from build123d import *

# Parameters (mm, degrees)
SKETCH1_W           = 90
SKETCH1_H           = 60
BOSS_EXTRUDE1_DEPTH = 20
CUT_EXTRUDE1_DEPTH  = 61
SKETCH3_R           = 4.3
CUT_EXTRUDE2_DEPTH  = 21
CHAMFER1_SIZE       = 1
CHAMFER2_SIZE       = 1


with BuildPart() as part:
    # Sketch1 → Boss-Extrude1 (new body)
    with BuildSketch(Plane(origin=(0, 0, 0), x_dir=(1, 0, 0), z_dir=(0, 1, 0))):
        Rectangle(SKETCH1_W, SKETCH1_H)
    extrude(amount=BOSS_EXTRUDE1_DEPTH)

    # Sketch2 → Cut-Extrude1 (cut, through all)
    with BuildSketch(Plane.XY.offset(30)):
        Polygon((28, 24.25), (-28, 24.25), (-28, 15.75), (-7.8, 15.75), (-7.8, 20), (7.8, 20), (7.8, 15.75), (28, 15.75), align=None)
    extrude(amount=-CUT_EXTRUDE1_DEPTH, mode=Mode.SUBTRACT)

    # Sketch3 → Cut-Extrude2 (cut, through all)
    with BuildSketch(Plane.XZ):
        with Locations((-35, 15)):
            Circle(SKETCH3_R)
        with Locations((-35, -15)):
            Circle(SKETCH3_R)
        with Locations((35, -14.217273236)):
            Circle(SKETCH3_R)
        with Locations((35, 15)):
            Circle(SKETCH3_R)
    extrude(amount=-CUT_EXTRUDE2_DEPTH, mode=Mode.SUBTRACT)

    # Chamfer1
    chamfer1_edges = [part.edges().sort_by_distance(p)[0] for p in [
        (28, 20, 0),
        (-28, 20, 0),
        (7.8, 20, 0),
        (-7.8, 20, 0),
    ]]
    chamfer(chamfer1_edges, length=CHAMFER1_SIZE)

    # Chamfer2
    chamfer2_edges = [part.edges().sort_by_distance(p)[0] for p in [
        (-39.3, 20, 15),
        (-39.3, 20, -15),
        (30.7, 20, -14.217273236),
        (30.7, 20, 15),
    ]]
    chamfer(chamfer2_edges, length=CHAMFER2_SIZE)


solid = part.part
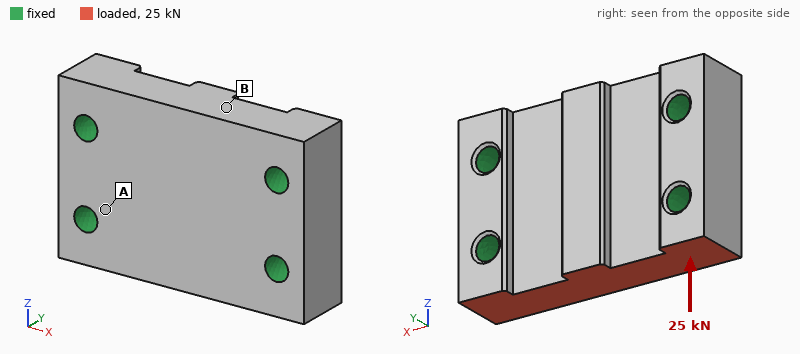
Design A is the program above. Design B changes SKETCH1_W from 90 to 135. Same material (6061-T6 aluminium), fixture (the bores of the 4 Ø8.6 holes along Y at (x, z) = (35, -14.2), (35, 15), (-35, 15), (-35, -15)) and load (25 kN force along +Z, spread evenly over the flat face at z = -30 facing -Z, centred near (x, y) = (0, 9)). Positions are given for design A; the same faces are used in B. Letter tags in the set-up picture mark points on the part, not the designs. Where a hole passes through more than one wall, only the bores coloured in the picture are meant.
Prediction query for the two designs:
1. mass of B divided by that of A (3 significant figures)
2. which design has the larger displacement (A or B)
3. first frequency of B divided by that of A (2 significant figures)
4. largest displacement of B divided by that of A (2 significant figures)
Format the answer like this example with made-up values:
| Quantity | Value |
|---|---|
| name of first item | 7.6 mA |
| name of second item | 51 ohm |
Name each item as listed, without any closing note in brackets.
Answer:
| Quantity | Value |
|---|---|
| mass of B divided by that of A | 1.58 |
| which design has the larger displacement | A |
| first frequency of B divided by that of A | 0.87 |
| largest displacement of B divided by that of A | 0.73 |
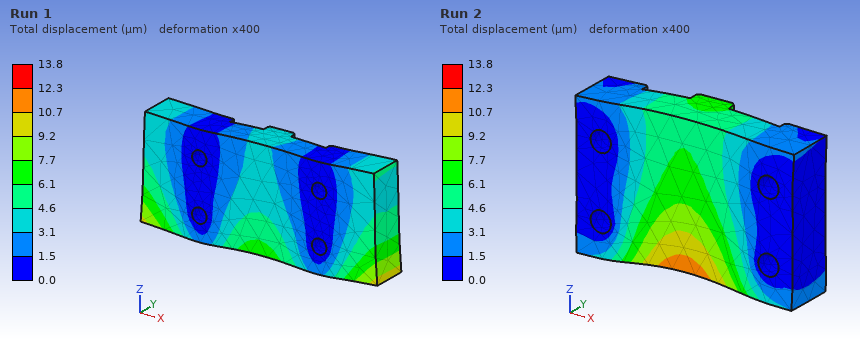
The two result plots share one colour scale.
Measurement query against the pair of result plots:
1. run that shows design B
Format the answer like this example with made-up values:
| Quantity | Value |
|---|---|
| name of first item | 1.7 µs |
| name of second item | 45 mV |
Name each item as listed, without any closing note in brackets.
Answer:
| Quantity | Value |
|---|---|
| run that shows design B | Run 1 |
